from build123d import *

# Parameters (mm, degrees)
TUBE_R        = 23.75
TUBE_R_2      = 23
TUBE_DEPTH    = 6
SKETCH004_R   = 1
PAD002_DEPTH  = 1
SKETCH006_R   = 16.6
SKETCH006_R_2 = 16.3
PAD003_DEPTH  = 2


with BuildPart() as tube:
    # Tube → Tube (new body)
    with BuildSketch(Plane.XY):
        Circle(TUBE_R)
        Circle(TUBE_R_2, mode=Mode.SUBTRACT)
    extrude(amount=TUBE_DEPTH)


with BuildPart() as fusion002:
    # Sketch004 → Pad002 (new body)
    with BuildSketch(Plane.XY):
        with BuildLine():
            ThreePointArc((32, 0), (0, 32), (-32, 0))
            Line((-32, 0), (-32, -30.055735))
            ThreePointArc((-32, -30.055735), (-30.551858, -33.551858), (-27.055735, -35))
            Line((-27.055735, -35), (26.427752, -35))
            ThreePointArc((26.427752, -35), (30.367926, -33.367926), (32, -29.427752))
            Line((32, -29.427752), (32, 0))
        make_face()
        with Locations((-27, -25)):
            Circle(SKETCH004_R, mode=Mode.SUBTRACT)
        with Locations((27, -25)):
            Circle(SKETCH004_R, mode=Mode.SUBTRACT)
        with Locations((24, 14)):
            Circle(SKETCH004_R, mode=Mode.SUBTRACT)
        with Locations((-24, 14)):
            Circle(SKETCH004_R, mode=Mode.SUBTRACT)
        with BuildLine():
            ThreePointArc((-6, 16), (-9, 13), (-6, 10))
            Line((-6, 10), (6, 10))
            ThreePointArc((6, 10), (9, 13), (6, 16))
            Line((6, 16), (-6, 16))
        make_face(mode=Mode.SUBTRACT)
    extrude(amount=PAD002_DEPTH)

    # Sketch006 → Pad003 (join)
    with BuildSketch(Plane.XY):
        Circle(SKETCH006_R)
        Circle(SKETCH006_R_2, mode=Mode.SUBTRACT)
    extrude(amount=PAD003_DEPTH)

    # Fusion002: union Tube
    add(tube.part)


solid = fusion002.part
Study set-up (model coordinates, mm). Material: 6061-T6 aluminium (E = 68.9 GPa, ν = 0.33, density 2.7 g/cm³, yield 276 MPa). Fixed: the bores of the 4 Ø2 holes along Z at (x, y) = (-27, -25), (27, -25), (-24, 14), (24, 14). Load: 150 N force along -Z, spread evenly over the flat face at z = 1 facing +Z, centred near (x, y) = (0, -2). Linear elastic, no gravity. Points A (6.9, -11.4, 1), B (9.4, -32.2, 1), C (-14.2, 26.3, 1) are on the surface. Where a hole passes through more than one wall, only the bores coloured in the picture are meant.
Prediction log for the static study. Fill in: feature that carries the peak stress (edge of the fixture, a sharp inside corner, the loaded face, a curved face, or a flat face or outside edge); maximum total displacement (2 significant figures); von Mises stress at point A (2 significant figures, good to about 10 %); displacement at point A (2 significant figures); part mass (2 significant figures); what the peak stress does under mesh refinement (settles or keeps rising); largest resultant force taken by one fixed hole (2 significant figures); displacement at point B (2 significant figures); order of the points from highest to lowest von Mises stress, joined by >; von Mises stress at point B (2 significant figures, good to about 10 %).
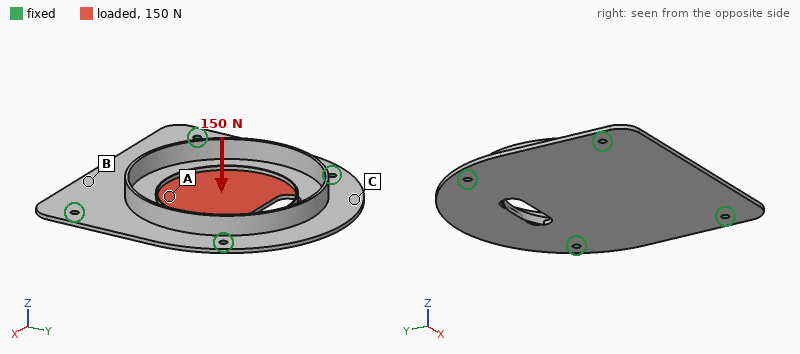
edge of the fixture
0.26 mm
30 MPa
0.19 mm
12 g
keeps rising
51 N
0.11 mm
A > B > C
17 MPa
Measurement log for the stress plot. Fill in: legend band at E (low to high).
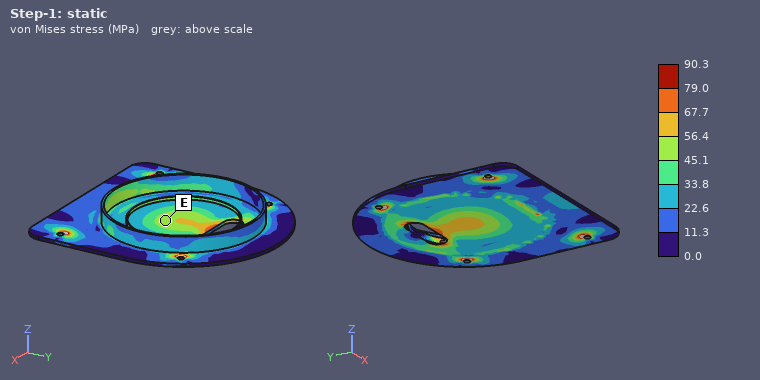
45.1 to 56.4 MPa
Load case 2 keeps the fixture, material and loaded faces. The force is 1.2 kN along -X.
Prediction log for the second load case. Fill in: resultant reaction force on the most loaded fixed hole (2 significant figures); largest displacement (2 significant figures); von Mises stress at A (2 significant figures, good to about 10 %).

340 N
21 µm
18 MPa
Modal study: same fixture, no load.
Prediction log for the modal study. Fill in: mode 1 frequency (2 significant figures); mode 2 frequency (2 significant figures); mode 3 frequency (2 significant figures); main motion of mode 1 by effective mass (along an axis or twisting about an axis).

1900 Hz
2400 Hz
3300 Hz
along Z
